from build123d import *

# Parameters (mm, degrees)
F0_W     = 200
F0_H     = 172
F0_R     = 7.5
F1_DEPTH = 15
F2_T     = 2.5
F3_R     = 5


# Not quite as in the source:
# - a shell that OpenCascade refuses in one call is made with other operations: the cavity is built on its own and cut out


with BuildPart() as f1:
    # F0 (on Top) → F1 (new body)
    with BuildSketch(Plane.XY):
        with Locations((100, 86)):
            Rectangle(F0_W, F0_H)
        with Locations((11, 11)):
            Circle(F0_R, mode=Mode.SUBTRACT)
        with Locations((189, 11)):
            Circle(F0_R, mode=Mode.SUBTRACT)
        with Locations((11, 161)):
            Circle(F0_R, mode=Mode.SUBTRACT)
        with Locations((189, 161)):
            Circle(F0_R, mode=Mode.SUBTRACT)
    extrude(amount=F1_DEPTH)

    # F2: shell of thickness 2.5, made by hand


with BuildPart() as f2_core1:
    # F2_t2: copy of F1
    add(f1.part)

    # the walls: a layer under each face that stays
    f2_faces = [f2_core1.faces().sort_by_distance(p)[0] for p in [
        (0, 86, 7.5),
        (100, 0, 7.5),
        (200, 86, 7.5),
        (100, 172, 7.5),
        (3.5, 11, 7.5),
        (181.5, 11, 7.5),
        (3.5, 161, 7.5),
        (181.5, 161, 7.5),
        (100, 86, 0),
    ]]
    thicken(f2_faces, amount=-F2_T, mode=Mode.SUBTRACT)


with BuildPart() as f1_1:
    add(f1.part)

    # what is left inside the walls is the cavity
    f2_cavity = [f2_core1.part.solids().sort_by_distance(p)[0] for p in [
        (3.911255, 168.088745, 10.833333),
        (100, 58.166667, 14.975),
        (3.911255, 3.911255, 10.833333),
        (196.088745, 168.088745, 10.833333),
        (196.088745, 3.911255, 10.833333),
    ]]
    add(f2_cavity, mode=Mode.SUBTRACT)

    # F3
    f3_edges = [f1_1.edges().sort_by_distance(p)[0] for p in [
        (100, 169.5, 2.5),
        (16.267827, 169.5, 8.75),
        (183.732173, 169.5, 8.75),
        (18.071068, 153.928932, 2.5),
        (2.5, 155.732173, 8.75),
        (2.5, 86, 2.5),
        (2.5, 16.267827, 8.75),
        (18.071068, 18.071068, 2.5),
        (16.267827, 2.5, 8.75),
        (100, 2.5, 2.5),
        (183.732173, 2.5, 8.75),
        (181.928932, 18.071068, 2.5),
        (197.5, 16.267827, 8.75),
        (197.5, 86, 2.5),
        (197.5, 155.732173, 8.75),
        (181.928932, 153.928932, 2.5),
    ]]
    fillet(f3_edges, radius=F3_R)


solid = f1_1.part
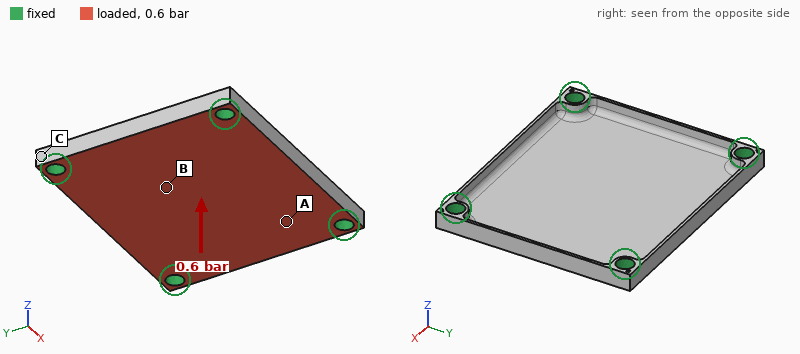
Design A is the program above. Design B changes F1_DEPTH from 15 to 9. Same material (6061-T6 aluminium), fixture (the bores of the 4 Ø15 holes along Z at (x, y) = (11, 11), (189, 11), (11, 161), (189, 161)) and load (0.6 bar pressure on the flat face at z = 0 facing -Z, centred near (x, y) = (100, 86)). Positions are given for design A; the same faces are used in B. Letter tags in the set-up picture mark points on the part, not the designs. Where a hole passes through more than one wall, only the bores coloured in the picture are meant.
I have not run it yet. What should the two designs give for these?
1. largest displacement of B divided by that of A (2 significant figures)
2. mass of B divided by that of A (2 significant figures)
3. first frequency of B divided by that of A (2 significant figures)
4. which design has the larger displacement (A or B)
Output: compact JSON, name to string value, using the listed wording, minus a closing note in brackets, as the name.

{"largest displacement of B divided by that of A": "1.1", "mass of B divided by that of A": "0.88", "first frequency of B divided by that of A": "0.95", "which design has the larger displacement": "B"}
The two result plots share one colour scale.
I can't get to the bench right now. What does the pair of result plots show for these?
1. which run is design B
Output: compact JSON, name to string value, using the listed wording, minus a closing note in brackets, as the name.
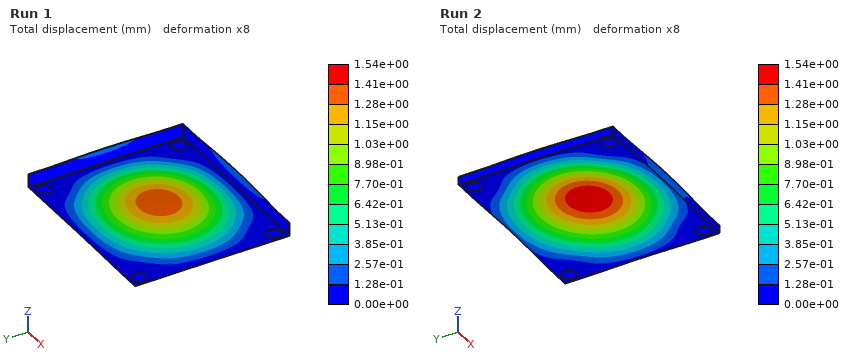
{"which run is design B": "Run 2"}
